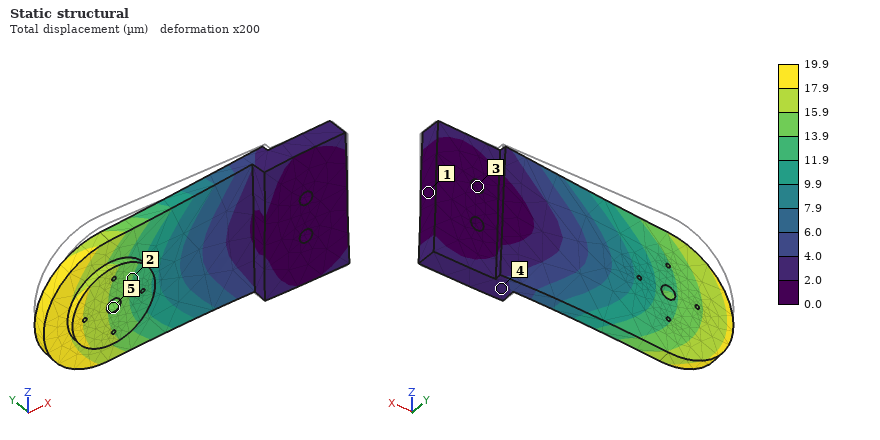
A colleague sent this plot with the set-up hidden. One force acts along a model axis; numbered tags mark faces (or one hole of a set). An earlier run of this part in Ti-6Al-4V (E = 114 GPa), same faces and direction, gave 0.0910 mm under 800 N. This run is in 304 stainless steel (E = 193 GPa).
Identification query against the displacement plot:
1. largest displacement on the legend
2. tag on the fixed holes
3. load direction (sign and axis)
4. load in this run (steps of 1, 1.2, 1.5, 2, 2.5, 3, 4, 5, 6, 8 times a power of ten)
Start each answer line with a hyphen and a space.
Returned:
- 19.9 µm
- 3
- -Z
- 300 N
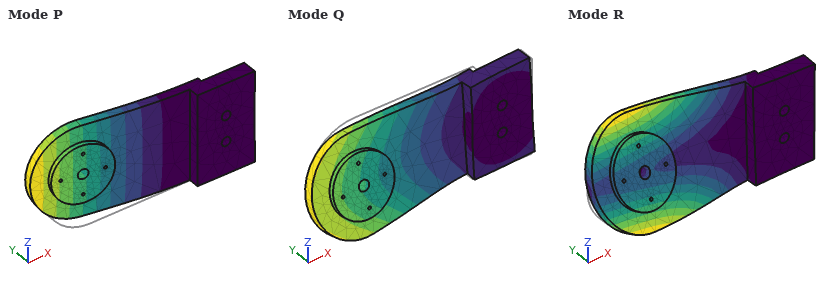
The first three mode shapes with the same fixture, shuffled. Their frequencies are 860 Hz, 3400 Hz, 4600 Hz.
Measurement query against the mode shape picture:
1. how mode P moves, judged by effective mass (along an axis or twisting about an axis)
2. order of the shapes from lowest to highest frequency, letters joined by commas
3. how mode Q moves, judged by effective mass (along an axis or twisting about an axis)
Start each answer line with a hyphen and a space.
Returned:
- along Y
- P, R, Q
- along Z
